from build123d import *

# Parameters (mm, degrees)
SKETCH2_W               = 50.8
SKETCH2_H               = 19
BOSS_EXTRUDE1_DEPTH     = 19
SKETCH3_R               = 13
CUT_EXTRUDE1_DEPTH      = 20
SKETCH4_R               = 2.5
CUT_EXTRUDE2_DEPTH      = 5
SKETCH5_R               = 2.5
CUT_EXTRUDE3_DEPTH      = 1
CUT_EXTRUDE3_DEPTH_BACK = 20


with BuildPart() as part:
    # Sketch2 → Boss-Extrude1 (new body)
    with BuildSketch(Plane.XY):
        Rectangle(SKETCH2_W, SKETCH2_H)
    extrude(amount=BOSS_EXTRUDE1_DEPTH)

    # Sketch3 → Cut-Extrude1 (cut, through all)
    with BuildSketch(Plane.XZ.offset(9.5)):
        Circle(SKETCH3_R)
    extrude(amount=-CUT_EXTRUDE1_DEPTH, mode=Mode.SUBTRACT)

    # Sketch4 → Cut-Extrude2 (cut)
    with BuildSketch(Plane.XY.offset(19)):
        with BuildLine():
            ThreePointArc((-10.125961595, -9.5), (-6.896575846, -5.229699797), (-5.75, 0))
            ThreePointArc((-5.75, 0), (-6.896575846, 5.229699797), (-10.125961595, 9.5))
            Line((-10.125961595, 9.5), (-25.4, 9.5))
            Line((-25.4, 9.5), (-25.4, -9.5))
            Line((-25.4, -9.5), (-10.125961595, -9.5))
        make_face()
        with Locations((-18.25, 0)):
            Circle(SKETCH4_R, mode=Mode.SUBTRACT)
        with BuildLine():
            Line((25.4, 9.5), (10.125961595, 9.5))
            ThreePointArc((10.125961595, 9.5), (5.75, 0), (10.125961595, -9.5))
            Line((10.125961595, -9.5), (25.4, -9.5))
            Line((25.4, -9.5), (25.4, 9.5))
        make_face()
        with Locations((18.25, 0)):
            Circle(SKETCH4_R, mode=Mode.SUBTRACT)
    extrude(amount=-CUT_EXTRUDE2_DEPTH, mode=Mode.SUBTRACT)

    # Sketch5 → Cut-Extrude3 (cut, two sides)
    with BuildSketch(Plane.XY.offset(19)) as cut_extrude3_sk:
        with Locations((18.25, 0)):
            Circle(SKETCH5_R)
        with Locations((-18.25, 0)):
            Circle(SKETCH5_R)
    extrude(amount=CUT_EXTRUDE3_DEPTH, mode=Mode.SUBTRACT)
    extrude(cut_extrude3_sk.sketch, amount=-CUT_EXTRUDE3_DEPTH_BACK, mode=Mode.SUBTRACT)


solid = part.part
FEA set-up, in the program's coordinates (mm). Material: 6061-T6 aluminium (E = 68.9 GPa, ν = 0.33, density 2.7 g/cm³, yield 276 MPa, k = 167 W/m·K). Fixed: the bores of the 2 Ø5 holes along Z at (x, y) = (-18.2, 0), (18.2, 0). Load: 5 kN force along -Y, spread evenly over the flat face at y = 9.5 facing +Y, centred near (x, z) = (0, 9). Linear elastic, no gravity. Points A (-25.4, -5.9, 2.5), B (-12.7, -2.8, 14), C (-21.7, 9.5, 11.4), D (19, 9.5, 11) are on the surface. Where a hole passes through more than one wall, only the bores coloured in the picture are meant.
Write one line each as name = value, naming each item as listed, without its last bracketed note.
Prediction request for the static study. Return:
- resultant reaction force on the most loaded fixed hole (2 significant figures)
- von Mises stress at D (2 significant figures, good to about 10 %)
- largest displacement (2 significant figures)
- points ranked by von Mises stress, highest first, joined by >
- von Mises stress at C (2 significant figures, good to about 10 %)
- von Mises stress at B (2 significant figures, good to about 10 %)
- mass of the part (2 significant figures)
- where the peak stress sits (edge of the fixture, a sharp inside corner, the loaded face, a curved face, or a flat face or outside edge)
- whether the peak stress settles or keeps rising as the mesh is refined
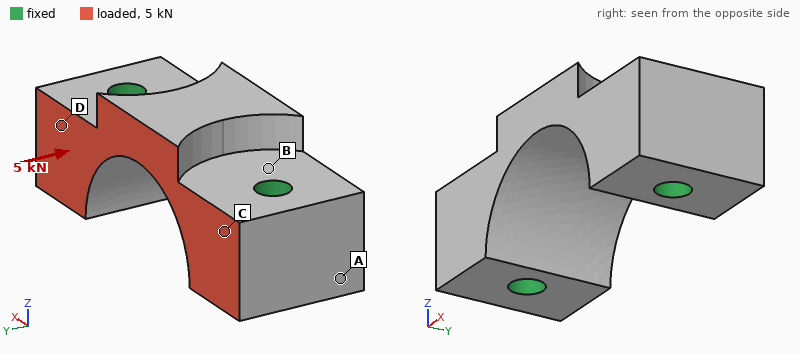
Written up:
resultant reaction force on the most loaded fixed hole = 2.5 kN
von Mises stress at D = 17 MPa
largest displacement = 21 µm
points ranked by von Mises stress, highest first, joined by > = B > D > C > A
von Mises stress at C = 12 MPa
von Mises stress at B = 24 MPa
mass of the part = 25 g
where the peak stress sits = edge of the fixture
whether the peak stress settles or keeps rising as the mesh is refined = keeps rising
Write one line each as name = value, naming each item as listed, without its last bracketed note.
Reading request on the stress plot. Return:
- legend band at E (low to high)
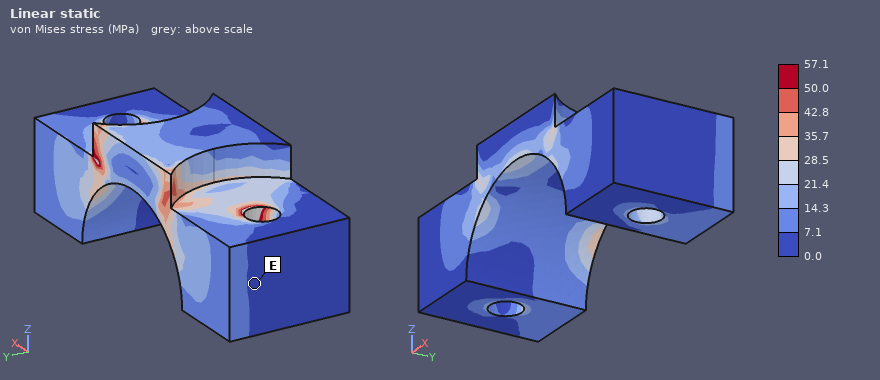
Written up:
legend band at E = 0.0 to 7.1 MPa
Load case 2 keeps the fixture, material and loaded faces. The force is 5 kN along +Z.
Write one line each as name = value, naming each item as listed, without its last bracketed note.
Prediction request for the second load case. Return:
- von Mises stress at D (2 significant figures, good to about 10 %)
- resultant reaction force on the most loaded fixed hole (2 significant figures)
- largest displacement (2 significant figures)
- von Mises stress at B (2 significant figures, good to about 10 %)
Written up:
von Mises stress at D = 21 MPa
resultant reaction force on the most loaded fixed hole = 2.6 kN
largest displacement = 28 µm
von Mises stress at B = 24 MPa
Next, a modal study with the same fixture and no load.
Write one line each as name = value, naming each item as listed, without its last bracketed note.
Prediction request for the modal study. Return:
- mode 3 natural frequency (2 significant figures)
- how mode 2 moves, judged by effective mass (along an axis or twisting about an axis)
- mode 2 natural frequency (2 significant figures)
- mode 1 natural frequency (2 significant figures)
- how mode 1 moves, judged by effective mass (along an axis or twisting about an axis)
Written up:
mode 3 natural frequency = 44 kHz
how mode 2 moves, judged by effective mass = along Z
mode 2 natural frequency = 33 kHz
mode 1 natural frequency = 22 kHz
how mode 1 moves, judged by effective mass = along Y
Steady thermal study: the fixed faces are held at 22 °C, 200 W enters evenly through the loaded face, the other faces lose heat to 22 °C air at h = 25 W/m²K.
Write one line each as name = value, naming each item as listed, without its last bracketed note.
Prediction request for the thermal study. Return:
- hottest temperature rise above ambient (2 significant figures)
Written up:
hottest temperature rise above ambient = 52 K
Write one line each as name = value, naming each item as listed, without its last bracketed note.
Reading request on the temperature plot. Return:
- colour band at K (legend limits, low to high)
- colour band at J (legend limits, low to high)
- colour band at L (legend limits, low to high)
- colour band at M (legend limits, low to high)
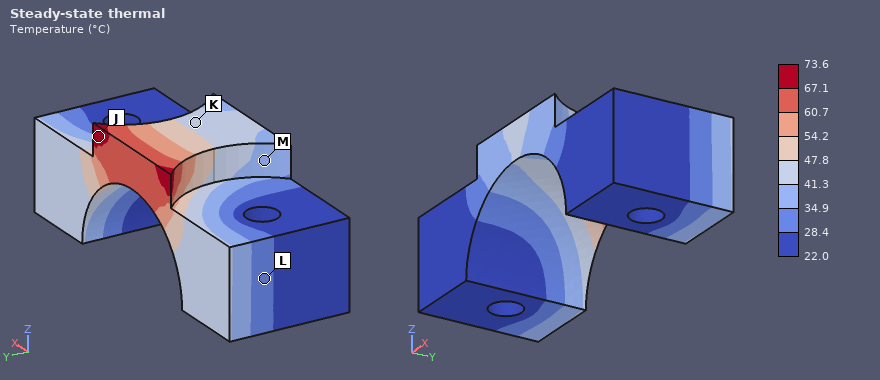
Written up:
colour band at K = 41.3 to 47.8 °C
colour band at J = 67.1 to 73.6 °C
colour band at L = 28.4 to 34.9 °C
colour band at M = 34.9 to 41.3 °C
